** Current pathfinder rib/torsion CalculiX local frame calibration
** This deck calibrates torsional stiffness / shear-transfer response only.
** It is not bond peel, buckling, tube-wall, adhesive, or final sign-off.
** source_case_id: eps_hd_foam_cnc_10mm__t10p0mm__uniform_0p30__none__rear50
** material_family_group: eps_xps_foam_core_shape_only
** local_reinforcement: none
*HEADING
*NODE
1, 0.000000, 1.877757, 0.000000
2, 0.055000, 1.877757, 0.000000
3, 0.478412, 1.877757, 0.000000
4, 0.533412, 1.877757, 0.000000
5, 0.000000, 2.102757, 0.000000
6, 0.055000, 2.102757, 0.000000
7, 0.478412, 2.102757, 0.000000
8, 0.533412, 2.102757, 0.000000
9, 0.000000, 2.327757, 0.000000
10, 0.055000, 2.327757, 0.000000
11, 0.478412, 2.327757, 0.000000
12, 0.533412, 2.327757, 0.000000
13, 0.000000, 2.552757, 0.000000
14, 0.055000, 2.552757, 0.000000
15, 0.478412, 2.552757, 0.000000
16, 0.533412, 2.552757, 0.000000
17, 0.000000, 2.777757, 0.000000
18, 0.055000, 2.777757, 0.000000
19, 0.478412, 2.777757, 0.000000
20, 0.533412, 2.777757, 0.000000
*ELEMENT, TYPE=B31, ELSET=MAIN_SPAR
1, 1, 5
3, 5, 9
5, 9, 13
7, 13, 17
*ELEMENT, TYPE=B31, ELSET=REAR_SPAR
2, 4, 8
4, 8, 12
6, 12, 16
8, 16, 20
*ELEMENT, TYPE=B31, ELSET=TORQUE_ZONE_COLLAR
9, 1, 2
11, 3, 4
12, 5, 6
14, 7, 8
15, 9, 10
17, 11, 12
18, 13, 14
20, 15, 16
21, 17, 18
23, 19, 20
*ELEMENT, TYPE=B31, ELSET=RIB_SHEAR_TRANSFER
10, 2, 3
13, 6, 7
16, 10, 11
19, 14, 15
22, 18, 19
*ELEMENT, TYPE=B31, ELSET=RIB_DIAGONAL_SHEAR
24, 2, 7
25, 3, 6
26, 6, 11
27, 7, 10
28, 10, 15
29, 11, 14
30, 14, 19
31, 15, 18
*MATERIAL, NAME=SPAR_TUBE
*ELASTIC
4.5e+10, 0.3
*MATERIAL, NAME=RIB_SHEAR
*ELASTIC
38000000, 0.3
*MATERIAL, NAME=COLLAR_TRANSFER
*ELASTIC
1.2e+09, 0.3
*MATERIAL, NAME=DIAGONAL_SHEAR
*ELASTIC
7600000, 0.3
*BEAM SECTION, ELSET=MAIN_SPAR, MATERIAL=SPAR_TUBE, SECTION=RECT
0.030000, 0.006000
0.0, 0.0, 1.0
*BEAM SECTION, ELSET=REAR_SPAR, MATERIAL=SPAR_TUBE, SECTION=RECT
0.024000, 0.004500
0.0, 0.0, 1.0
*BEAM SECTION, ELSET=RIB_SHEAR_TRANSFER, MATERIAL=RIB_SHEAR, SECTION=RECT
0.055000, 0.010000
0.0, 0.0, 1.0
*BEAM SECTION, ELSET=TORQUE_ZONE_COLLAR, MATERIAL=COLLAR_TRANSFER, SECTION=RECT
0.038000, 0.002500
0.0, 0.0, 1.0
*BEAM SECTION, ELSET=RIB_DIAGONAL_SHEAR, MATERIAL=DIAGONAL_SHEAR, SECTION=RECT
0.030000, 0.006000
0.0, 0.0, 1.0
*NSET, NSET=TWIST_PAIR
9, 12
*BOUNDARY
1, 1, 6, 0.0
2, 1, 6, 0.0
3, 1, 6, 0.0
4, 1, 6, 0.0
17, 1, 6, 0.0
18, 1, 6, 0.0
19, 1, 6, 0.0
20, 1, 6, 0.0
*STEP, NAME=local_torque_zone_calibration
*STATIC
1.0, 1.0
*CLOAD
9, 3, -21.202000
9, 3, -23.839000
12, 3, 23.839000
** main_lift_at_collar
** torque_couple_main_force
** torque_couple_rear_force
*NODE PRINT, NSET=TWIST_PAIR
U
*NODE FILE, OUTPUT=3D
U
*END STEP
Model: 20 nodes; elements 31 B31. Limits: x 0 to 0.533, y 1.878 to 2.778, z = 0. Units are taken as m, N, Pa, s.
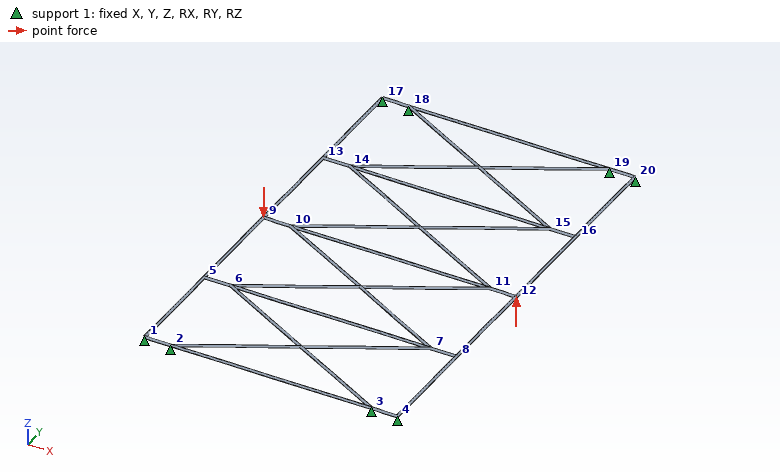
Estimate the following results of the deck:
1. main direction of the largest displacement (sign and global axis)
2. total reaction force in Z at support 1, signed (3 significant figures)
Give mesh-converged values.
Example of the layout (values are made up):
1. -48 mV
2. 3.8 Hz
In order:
1. +Z
2. 21.2 N
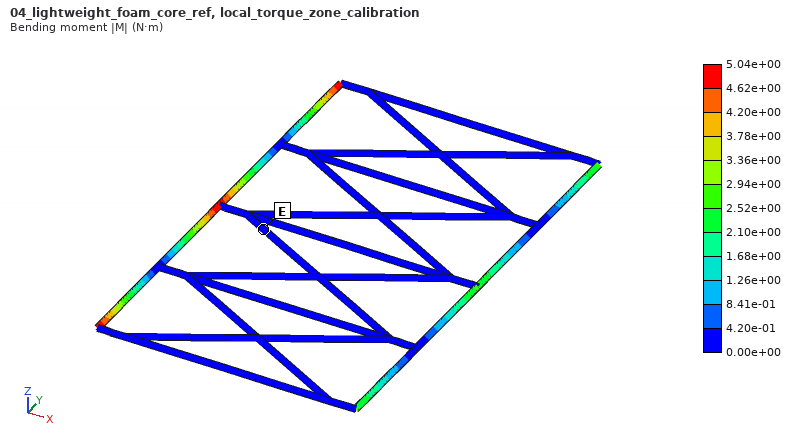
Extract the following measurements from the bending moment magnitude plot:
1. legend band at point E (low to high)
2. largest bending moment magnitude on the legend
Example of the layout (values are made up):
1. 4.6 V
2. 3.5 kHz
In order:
1. 0.00e+00 to 4.20e-01 N·m
2. 5.04e+00 N·m
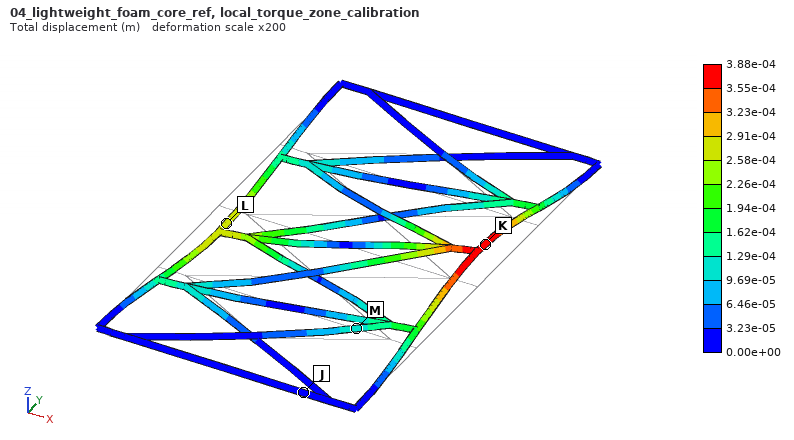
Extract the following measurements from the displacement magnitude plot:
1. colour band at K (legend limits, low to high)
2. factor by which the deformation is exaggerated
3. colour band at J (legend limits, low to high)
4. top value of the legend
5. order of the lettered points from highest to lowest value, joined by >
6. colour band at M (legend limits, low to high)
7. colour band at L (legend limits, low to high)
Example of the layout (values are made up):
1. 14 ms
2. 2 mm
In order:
1. 3.55e-04 to 3.88e-04 m
2. 200
3. 0.00e+00 to 3.23e-05 m
4. 3.88e-04 m
5. K > L > M > J
6. 9.69e-05 to 1.29e-04 m
7. 2.58e-04 to 2.91e-04 m
